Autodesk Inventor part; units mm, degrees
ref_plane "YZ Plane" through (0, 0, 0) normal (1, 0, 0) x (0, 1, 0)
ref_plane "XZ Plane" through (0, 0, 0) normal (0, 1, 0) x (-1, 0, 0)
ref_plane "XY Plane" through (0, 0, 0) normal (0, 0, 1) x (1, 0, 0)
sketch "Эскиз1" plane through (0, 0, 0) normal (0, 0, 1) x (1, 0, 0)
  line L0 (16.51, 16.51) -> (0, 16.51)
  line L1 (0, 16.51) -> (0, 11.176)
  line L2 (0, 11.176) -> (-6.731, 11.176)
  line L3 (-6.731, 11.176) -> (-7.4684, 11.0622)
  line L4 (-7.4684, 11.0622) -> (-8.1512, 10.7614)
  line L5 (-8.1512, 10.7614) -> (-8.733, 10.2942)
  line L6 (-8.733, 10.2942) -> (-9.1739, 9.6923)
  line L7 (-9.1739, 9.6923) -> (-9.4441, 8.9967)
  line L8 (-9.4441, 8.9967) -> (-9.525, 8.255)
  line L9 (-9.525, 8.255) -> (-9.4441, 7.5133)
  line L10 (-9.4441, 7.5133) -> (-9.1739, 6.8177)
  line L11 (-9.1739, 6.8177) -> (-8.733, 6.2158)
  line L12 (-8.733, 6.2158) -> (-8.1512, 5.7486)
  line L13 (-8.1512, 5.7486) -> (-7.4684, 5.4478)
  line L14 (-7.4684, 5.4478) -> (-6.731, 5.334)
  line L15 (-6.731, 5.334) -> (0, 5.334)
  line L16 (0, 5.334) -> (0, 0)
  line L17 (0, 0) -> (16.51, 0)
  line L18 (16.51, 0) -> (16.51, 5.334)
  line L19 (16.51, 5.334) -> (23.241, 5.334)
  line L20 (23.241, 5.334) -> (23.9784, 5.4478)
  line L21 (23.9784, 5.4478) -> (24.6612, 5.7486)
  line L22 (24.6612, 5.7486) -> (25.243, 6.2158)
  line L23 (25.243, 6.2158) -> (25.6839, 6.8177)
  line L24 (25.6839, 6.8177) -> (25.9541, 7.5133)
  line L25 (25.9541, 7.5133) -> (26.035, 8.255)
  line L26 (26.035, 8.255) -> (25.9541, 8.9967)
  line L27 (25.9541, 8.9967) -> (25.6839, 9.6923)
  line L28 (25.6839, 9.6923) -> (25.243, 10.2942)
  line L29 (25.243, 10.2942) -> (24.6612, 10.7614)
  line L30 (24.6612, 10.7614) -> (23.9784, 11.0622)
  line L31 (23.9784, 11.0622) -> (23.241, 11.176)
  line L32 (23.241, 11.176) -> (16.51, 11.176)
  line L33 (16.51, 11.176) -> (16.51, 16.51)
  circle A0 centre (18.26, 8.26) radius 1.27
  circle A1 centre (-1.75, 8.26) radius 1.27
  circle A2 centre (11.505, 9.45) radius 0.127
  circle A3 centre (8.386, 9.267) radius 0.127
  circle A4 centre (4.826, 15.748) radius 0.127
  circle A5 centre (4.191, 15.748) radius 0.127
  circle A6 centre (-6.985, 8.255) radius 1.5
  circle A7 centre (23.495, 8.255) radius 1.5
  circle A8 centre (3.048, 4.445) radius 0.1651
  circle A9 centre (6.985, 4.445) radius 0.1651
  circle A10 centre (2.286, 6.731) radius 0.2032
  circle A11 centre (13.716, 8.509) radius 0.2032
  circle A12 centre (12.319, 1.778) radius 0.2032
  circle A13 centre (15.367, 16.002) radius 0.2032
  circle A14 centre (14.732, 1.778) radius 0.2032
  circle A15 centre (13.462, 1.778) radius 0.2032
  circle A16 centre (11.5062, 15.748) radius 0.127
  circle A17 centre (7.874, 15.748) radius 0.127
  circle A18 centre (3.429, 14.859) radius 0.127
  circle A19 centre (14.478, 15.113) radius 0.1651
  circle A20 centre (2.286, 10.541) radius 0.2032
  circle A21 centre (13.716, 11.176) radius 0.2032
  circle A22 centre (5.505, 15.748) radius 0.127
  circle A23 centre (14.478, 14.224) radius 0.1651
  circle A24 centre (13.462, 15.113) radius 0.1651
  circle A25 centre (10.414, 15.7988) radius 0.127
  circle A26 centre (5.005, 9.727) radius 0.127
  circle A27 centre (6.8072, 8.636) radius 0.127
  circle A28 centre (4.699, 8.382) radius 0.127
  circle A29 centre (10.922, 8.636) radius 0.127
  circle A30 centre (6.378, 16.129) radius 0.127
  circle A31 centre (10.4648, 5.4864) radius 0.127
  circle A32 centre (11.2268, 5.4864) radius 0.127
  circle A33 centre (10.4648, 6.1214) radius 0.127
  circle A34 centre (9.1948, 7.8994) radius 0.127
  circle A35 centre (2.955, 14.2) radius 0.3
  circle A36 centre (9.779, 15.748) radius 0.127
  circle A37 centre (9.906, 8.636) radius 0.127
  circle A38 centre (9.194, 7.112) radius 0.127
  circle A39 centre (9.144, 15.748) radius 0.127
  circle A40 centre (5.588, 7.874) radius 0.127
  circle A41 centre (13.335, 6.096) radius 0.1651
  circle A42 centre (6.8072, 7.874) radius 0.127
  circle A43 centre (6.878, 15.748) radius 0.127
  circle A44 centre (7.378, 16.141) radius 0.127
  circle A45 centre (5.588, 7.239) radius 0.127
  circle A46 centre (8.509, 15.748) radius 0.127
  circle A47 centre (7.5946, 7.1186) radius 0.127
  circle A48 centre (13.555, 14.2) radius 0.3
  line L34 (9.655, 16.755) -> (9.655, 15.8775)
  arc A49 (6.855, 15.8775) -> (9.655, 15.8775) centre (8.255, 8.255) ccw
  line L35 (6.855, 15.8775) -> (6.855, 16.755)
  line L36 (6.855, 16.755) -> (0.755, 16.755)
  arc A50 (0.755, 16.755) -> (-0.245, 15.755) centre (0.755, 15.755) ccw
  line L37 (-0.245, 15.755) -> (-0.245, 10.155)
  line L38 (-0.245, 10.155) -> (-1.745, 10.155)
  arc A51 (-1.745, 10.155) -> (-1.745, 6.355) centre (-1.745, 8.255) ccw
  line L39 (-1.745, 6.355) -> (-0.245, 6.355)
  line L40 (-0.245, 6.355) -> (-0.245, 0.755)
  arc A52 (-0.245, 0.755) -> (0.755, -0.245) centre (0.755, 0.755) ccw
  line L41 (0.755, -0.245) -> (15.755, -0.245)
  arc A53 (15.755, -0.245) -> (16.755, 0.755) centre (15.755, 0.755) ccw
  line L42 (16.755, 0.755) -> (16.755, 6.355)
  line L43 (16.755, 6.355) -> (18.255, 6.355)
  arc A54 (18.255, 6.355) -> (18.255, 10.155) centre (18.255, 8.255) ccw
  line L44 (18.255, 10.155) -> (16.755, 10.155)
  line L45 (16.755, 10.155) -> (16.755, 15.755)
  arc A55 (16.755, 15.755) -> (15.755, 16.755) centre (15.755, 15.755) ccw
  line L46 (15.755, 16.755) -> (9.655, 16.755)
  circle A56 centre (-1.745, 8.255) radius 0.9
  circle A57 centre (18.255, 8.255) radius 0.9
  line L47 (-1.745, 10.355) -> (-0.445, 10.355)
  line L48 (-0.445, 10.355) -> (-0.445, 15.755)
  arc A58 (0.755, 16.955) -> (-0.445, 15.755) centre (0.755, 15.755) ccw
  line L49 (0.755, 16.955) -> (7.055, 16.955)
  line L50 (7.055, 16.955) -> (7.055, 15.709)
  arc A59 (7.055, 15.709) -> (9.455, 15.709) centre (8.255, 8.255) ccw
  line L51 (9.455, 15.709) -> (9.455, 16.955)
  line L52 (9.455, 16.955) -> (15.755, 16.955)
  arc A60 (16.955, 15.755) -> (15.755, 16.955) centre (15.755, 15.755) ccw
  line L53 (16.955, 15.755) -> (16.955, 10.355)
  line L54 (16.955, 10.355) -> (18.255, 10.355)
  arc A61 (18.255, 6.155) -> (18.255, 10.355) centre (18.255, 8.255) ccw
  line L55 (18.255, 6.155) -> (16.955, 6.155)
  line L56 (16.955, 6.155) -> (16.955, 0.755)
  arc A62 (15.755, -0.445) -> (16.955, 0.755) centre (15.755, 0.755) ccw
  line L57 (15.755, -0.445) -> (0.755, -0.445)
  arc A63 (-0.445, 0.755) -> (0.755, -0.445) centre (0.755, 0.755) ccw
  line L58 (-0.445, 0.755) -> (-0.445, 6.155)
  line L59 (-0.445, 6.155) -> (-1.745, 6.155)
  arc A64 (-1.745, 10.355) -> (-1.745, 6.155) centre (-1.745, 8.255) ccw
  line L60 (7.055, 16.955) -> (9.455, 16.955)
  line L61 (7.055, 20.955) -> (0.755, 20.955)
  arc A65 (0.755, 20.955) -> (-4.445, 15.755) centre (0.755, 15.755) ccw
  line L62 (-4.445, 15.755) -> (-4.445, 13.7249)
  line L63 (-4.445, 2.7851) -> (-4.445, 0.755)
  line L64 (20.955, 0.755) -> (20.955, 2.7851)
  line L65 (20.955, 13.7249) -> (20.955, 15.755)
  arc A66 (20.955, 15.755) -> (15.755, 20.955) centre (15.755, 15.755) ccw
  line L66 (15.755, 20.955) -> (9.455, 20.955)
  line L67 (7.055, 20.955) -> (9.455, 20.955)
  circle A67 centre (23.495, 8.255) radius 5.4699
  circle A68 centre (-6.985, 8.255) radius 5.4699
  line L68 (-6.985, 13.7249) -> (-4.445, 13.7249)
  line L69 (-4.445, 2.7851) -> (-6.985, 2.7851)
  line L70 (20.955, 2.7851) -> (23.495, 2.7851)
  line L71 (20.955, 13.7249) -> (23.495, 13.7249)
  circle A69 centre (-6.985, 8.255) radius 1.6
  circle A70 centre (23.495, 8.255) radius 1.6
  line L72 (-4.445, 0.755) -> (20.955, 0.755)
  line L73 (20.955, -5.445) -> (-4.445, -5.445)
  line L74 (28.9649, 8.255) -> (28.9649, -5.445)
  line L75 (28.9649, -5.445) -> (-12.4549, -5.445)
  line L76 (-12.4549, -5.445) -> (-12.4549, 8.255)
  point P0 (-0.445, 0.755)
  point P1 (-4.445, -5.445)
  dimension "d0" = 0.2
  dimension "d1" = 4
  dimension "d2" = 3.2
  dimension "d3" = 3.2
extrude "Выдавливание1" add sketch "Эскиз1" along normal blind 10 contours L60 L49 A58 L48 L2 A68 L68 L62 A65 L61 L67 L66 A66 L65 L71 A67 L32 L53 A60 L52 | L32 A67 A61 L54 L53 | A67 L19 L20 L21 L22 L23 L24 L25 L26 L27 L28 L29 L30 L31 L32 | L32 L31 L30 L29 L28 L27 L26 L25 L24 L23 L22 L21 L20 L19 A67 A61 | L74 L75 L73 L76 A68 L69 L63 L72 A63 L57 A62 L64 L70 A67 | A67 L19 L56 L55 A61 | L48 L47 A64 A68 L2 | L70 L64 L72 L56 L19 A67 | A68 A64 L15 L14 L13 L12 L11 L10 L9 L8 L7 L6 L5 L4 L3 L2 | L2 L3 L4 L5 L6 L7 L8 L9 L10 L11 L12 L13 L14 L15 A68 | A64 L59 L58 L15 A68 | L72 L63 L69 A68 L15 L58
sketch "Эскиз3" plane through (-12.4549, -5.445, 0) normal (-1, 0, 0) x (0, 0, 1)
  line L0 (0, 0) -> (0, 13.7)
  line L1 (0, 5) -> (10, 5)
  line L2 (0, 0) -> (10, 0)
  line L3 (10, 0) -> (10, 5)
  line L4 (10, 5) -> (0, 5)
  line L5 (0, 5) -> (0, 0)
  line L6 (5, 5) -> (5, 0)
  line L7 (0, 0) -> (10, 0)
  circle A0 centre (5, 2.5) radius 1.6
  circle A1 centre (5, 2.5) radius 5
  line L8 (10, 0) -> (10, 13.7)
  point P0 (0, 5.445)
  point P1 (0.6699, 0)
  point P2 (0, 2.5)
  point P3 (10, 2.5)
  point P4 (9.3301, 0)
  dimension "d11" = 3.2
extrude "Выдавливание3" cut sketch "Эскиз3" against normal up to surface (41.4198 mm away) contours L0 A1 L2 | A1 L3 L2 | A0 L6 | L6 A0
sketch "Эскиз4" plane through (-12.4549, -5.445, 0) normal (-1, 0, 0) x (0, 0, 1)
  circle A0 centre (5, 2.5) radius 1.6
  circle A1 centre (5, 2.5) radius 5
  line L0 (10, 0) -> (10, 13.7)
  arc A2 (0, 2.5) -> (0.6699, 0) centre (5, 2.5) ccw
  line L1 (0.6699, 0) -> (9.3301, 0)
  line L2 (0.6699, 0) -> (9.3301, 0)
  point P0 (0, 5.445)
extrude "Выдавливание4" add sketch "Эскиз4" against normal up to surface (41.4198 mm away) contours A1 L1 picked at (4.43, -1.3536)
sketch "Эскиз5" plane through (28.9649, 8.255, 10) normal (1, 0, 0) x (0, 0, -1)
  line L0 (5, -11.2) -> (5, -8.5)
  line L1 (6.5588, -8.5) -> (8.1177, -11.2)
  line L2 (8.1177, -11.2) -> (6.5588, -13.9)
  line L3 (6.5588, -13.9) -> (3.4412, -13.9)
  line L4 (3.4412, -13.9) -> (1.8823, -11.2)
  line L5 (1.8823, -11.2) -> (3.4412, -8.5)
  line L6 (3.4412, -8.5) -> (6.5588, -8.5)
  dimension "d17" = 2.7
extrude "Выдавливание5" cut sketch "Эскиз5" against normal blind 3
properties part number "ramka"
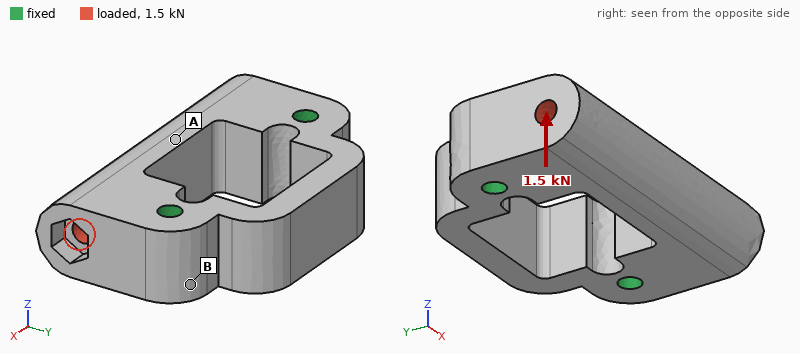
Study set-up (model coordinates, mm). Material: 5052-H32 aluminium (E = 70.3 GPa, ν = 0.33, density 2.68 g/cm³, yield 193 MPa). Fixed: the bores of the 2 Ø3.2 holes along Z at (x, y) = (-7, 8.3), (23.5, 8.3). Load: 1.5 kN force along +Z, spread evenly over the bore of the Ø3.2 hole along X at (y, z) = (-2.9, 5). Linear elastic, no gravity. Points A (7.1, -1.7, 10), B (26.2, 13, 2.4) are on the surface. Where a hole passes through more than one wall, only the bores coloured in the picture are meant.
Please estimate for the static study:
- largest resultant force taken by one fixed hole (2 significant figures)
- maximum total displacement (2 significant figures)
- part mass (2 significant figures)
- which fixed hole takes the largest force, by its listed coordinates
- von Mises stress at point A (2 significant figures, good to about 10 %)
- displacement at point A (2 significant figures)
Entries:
810 N
20 µm
17 g
(-7, 8.3)
23 MPa
15 µm
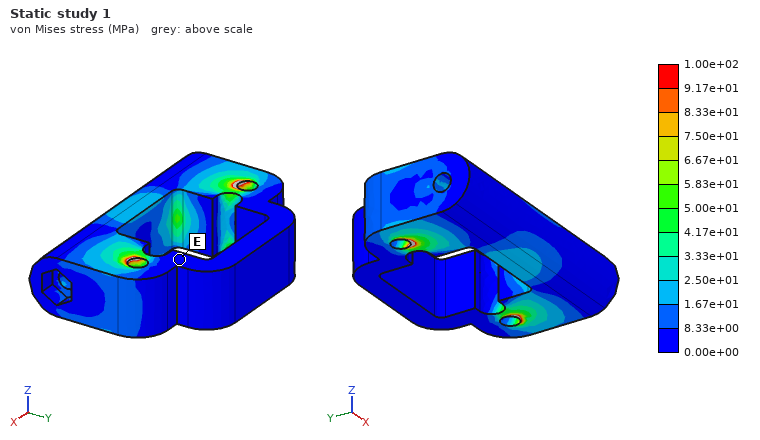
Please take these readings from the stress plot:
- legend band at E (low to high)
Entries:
0.00e+00 to 8.33e+00 MPa
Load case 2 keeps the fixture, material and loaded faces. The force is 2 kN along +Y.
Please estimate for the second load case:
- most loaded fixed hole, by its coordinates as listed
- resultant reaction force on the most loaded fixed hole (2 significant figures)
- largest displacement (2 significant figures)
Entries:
(-7, 8.3)
1.1 kN
7.7 µm
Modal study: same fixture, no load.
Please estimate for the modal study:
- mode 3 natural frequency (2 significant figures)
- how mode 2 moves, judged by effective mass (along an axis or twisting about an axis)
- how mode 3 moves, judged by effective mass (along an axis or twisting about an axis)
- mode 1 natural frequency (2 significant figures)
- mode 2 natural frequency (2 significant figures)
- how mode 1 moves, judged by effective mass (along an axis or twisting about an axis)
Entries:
23 kHz
along X
along Z
19 kHz
22 kHz
along Z
